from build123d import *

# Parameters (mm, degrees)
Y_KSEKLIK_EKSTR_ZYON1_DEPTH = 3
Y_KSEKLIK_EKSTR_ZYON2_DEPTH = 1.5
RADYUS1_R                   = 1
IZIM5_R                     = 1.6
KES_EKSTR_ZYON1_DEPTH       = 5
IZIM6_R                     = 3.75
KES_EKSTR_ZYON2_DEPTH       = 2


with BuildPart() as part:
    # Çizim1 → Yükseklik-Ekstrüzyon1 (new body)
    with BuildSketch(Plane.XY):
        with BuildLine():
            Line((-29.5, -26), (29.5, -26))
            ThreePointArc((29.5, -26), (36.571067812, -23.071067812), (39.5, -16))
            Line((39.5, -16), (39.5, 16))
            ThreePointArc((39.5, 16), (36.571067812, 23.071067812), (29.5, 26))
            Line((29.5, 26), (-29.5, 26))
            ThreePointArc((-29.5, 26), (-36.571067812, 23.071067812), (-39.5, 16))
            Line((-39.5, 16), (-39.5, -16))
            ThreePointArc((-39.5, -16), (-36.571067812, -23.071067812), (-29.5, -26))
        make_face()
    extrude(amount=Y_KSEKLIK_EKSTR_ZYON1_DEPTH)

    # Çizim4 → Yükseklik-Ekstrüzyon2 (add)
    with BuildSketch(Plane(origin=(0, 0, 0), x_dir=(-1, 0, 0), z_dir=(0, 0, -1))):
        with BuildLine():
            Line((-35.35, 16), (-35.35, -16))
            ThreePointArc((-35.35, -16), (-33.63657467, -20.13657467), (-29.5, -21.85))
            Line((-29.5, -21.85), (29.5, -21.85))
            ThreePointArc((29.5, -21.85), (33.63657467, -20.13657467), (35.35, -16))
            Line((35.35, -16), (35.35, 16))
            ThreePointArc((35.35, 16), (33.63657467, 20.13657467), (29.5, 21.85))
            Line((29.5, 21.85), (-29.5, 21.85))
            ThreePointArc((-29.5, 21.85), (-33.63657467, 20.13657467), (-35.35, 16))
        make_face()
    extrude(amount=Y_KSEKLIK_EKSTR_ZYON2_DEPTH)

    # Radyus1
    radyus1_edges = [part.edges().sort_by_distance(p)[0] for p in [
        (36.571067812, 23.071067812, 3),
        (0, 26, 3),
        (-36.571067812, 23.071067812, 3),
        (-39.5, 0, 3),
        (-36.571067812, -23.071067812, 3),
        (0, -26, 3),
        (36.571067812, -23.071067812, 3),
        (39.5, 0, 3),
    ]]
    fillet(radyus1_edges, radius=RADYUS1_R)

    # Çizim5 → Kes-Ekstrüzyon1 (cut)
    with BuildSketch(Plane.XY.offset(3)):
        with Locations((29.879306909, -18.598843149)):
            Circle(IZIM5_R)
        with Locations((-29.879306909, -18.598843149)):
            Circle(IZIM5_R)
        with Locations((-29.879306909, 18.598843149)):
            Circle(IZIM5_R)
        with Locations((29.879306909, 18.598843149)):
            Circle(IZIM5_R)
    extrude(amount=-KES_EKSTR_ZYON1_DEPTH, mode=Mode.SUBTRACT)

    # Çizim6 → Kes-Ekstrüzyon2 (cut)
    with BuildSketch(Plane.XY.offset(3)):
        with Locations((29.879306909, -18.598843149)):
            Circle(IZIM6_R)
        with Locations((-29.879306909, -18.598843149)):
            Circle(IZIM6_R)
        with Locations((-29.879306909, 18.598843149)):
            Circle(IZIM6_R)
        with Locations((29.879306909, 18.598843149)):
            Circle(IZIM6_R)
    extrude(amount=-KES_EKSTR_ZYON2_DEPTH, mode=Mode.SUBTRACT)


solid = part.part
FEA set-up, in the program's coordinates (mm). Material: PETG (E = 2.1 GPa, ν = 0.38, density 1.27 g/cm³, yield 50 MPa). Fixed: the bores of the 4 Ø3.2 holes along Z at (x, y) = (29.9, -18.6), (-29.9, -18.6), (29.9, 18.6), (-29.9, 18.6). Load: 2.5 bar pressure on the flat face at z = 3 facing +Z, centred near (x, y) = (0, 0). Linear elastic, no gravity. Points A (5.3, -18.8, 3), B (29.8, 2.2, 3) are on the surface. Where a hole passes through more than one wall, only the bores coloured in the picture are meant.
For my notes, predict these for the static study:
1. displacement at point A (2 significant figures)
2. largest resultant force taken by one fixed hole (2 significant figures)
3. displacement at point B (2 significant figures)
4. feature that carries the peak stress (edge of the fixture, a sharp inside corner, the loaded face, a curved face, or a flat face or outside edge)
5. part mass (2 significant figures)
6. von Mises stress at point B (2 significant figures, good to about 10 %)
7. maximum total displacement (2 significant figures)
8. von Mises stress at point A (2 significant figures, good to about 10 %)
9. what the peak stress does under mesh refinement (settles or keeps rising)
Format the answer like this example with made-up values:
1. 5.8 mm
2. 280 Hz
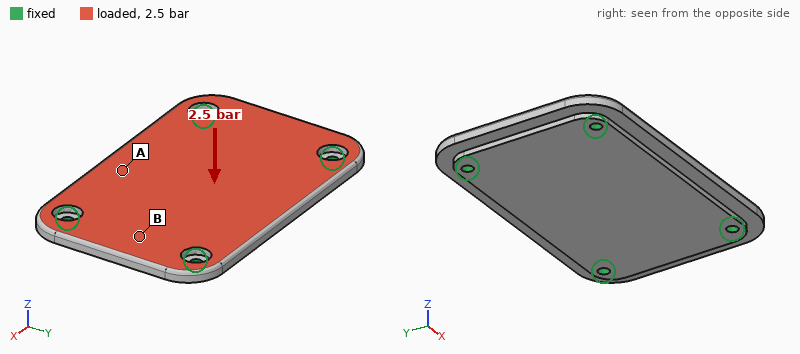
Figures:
1. 1.0 mm
2. 320 N
3. 0.25 mm
4. edge of the fixture
5. 21 g
6. 8.8 MPa
7. 1.1 mm
8. 17 MPa
9. keeps rising
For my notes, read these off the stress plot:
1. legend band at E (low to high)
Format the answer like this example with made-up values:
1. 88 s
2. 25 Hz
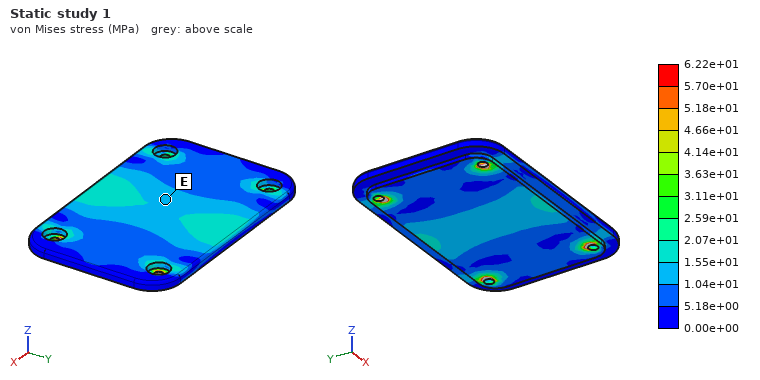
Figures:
1. 1.04e+01 to 1.55e+01 MPa
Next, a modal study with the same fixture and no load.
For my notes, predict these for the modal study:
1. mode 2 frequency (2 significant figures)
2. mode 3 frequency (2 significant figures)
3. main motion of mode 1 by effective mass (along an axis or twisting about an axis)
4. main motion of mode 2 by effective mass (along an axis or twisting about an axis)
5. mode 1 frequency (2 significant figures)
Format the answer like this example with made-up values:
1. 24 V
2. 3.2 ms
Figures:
1. 1700 Hz
2. 2700 Hz
3. along Z
4. twisting about X
5. 1100 Hz
